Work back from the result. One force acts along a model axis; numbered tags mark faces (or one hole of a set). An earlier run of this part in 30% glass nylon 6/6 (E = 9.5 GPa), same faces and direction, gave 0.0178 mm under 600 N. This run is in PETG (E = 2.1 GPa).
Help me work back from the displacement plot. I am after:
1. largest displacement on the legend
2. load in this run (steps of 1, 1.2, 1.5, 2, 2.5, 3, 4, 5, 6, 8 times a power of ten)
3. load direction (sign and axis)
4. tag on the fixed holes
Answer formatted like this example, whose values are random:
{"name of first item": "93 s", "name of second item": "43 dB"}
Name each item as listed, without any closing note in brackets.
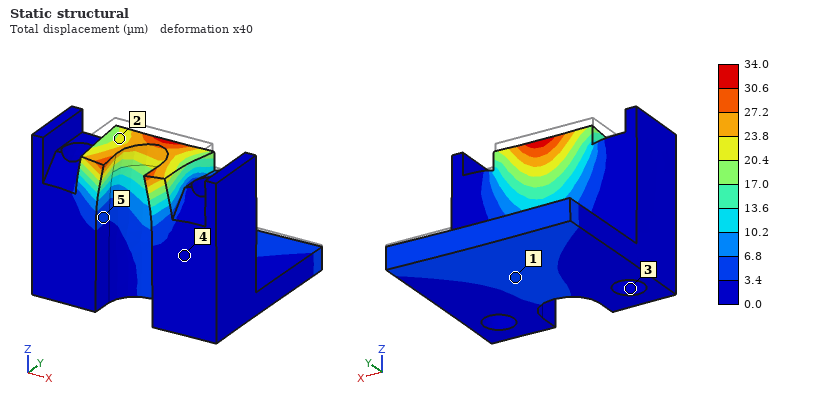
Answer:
{"largest displacement on the legend": "34.0 µm", "load in this run": "250 N", "load direction": "-Z", "tag on the fixed holes": "3"}
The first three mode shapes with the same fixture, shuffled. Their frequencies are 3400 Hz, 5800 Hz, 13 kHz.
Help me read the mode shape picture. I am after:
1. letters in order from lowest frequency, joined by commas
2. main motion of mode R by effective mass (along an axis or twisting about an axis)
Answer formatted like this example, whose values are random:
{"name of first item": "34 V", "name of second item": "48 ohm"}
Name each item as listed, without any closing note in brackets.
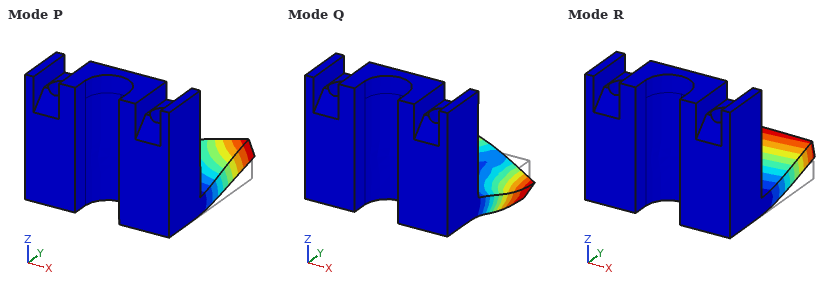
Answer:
{"letters in order from lowest frequency, joined by commas": "R, P, Q", "main motion of mode R by effective mass": "along Z"}
